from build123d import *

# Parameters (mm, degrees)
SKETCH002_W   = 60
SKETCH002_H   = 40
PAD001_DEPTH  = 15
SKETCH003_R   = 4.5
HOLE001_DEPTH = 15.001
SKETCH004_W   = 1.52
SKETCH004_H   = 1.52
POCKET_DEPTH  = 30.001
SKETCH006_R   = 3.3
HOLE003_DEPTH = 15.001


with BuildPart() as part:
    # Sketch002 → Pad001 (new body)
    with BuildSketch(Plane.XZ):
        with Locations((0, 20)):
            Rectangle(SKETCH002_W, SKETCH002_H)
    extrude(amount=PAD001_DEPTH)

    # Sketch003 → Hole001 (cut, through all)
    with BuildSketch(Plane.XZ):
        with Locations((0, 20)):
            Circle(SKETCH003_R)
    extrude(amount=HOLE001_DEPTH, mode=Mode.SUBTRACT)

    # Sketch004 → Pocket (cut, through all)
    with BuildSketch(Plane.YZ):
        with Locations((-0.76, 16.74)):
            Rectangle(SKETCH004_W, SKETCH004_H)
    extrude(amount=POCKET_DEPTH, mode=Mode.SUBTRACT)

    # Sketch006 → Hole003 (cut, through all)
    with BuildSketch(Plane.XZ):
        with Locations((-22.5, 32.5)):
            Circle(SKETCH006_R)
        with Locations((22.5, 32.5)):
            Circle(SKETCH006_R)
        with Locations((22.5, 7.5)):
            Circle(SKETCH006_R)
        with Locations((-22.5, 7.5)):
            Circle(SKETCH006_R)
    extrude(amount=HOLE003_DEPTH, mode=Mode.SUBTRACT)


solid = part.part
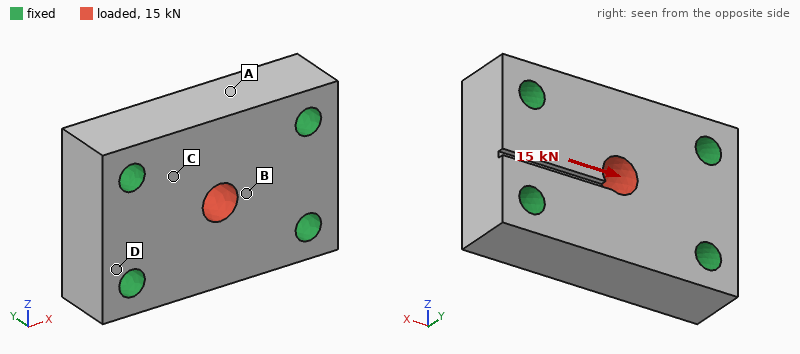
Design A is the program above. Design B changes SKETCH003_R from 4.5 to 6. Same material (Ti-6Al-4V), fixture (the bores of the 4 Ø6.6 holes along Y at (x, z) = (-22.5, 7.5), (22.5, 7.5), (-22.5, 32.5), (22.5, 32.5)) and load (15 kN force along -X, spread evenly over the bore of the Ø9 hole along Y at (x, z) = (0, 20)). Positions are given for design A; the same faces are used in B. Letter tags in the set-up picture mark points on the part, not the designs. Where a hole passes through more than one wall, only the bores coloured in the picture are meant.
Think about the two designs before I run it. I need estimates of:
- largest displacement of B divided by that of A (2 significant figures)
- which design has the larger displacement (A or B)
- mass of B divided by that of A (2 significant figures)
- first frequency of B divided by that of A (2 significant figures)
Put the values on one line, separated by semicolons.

0.80; A; 0.98; 1.0
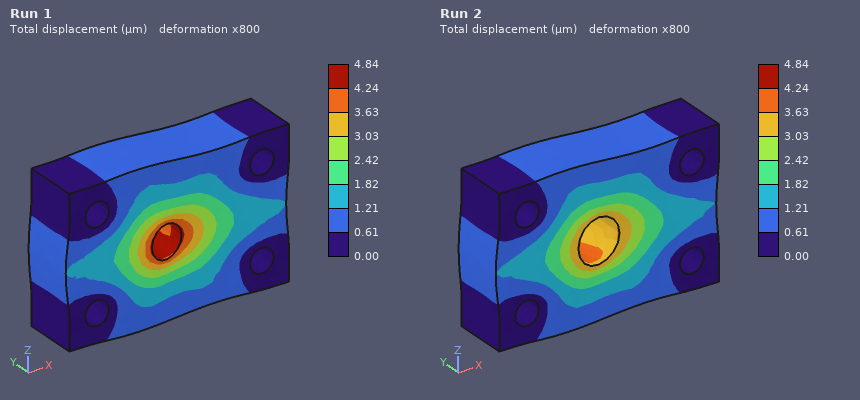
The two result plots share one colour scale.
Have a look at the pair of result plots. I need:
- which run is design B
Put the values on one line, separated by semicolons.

Run 2
